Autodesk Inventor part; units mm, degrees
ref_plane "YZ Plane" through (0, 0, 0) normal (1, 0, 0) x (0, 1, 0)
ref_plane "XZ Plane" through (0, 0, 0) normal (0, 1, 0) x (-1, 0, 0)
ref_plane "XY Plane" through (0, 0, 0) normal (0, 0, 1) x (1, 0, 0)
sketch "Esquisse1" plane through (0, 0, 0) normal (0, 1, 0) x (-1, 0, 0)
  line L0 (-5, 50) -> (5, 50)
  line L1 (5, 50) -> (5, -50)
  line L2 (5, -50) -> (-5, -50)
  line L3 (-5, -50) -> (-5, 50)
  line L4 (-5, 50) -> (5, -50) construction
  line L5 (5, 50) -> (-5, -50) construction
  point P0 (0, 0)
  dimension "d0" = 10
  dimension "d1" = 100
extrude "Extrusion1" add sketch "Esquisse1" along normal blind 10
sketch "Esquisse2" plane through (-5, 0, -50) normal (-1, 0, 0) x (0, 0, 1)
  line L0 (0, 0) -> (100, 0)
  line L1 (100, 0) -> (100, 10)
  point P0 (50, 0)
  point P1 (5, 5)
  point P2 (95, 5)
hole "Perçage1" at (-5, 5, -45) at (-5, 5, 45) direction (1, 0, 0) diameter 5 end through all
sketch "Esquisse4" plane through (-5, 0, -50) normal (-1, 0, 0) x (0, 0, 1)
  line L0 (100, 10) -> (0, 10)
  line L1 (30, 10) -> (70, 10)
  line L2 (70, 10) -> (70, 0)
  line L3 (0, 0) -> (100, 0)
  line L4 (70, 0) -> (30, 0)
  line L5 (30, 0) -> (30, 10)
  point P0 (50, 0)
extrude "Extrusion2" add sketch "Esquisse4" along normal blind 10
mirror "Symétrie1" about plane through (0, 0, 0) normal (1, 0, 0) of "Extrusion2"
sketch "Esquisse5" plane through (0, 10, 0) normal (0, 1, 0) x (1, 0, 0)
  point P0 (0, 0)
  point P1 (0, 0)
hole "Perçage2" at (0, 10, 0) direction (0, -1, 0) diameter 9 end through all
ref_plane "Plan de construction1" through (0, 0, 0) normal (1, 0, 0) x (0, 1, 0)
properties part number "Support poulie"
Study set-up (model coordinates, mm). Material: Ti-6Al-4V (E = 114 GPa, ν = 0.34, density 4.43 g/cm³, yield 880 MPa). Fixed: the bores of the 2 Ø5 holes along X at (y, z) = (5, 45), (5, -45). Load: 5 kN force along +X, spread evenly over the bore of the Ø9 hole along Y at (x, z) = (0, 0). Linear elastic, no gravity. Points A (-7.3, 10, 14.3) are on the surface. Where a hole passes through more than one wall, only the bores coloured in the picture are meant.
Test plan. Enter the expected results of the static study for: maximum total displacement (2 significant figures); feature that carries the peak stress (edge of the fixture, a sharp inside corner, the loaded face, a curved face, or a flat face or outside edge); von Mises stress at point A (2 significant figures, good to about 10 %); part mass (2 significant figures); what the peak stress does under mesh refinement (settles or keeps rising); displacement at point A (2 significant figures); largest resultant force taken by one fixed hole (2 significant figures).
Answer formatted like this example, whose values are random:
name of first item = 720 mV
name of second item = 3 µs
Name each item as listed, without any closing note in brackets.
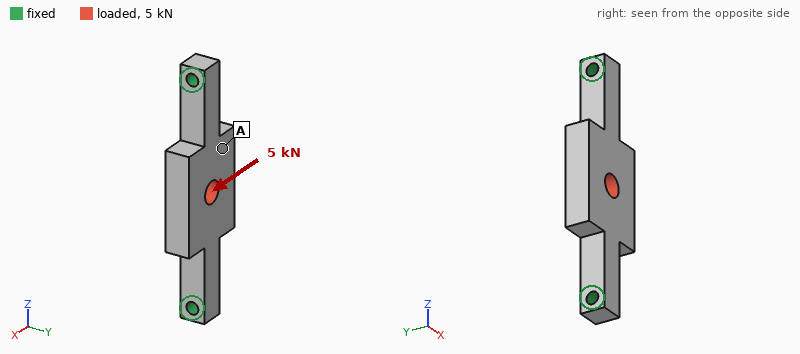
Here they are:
maximum total displacement = 68 µm
feature that carries the peak stress = edge of the fixture
von Mises stress at point A = 46 MPa
part mass = 75 g
what the peak stress does under mesh refinement = keeps rising
displacement at point A = 62 µm
largest resultant force taken by one fixed hole = 2.5 kN
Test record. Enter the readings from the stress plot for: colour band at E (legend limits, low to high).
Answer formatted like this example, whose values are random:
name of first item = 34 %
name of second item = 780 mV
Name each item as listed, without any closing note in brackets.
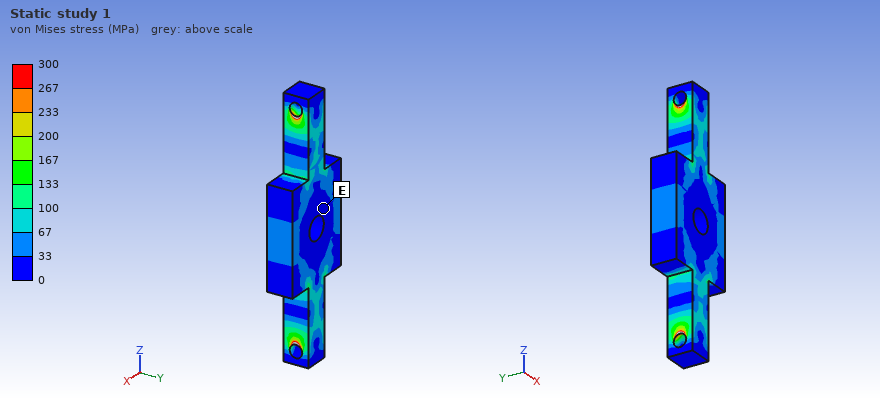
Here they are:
colour band at E = 0 to 33 MPa
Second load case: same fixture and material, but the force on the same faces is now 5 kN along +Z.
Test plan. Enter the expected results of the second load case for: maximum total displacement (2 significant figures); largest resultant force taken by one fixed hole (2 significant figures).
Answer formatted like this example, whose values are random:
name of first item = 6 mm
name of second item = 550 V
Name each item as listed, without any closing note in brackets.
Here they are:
maximum total displacement = 8.1 µm
largest resultant force taken by one fixed hole = 2.5 kN
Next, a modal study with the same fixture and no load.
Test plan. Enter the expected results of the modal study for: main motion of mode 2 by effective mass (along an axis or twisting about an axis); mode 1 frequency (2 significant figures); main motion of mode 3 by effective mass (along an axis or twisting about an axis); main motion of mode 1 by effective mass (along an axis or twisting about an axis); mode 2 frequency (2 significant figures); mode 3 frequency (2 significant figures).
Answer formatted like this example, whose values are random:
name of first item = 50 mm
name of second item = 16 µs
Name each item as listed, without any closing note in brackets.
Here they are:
main motion of mode 2 by effective mass = twisting about Z
mode 1 frequency = 4200 Hz
main motion of mode 3 by effective mass = along X
main motion of mode 1 by effective mass = along Y
mode 2 frequency = 5100 Hz
mode 3 frequency = 6000 Hz
